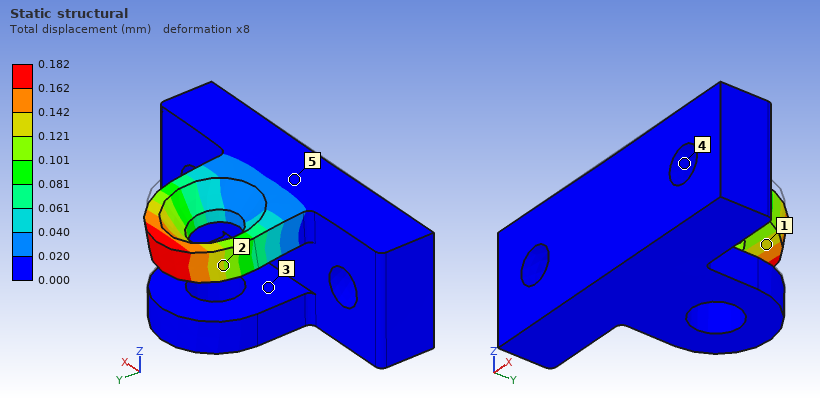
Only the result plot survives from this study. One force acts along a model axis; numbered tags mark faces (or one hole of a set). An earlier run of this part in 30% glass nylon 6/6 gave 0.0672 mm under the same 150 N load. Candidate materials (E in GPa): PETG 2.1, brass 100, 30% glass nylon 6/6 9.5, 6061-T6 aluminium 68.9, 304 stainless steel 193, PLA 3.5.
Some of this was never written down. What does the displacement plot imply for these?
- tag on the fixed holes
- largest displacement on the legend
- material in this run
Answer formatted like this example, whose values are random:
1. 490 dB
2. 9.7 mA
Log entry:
1. 4
2. 0.182 mm
3. PLA
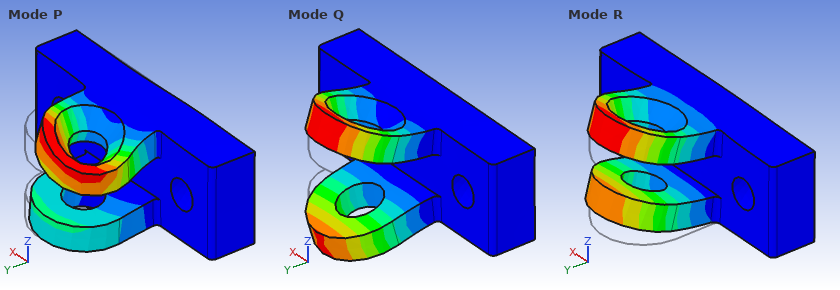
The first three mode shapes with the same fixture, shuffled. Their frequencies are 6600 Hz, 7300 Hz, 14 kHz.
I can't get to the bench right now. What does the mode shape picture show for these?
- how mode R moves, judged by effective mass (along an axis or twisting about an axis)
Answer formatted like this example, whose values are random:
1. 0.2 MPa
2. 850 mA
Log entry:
1. along Z
